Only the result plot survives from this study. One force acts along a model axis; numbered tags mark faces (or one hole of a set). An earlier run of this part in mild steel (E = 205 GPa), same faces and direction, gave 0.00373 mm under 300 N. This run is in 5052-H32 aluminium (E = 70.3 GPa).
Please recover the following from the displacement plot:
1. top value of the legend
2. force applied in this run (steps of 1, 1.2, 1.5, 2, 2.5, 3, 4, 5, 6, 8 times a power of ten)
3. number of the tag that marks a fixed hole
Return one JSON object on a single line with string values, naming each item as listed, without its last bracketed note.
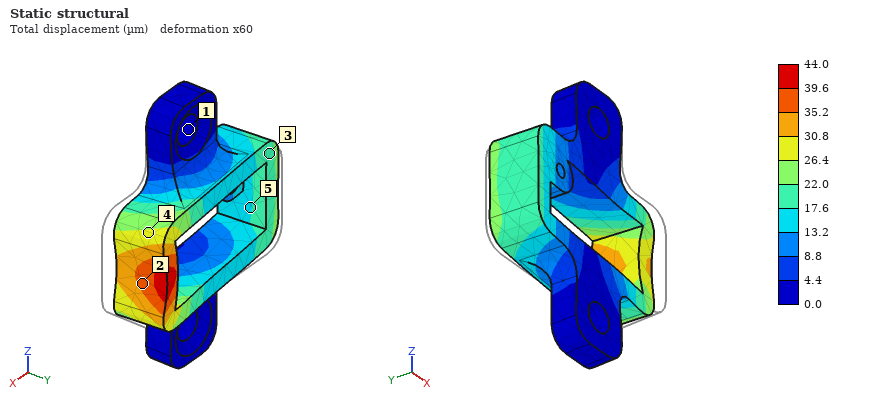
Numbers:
{"top value of the legend": "44.0 µm", "force applied in this run": "1.2 kN", "number of the tag that marks a fixed hole": "1"}
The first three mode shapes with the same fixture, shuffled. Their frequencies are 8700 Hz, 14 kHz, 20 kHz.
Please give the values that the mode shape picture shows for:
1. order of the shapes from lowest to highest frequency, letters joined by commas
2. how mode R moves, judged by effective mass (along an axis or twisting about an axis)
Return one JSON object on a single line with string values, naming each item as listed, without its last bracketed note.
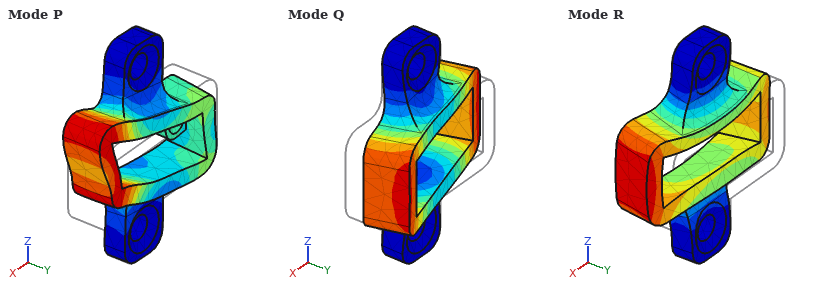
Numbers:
{"order of the shapes from lowest to highest frequency, letters joined by commas": "Q, R, P", "how mode R moves, judged by effective mass": "along Y"}
